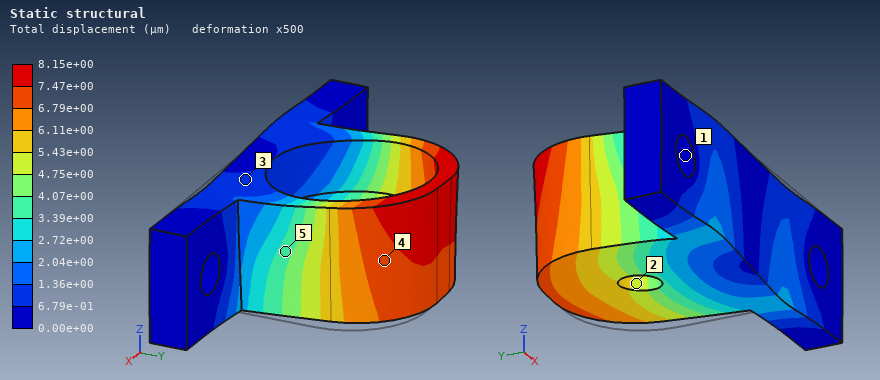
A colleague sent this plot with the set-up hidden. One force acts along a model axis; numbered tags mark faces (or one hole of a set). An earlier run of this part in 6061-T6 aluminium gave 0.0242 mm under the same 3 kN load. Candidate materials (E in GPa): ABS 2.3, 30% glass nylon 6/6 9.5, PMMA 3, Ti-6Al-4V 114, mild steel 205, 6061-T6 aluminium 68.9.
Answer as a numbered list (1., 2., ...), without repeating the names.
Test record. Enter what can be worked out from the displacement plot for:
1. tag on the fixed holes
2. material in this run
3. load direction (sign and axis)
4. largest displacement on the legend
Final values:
1. 1
2. mild steel
3. -X
4. 8.15e+00 µm
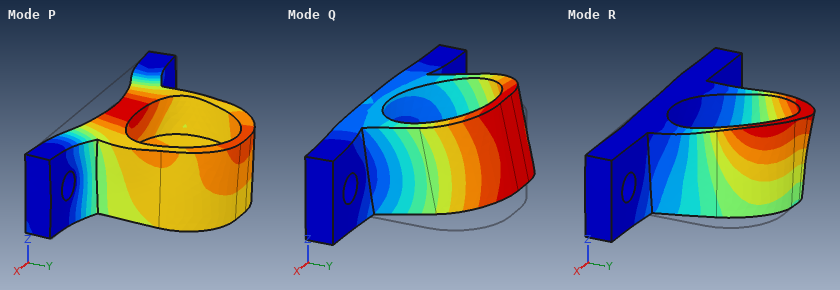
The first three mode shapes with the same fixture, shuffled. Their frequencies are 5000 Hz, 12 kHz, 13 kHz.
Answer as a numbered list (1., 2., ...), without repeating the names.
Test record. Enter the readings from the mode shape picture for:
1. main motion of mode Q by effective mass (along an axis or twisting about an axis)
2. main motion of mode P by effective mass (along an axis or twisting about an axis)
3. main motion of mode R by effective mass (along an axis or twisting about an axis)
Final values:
1. along Z
2. along Y
3. along X
